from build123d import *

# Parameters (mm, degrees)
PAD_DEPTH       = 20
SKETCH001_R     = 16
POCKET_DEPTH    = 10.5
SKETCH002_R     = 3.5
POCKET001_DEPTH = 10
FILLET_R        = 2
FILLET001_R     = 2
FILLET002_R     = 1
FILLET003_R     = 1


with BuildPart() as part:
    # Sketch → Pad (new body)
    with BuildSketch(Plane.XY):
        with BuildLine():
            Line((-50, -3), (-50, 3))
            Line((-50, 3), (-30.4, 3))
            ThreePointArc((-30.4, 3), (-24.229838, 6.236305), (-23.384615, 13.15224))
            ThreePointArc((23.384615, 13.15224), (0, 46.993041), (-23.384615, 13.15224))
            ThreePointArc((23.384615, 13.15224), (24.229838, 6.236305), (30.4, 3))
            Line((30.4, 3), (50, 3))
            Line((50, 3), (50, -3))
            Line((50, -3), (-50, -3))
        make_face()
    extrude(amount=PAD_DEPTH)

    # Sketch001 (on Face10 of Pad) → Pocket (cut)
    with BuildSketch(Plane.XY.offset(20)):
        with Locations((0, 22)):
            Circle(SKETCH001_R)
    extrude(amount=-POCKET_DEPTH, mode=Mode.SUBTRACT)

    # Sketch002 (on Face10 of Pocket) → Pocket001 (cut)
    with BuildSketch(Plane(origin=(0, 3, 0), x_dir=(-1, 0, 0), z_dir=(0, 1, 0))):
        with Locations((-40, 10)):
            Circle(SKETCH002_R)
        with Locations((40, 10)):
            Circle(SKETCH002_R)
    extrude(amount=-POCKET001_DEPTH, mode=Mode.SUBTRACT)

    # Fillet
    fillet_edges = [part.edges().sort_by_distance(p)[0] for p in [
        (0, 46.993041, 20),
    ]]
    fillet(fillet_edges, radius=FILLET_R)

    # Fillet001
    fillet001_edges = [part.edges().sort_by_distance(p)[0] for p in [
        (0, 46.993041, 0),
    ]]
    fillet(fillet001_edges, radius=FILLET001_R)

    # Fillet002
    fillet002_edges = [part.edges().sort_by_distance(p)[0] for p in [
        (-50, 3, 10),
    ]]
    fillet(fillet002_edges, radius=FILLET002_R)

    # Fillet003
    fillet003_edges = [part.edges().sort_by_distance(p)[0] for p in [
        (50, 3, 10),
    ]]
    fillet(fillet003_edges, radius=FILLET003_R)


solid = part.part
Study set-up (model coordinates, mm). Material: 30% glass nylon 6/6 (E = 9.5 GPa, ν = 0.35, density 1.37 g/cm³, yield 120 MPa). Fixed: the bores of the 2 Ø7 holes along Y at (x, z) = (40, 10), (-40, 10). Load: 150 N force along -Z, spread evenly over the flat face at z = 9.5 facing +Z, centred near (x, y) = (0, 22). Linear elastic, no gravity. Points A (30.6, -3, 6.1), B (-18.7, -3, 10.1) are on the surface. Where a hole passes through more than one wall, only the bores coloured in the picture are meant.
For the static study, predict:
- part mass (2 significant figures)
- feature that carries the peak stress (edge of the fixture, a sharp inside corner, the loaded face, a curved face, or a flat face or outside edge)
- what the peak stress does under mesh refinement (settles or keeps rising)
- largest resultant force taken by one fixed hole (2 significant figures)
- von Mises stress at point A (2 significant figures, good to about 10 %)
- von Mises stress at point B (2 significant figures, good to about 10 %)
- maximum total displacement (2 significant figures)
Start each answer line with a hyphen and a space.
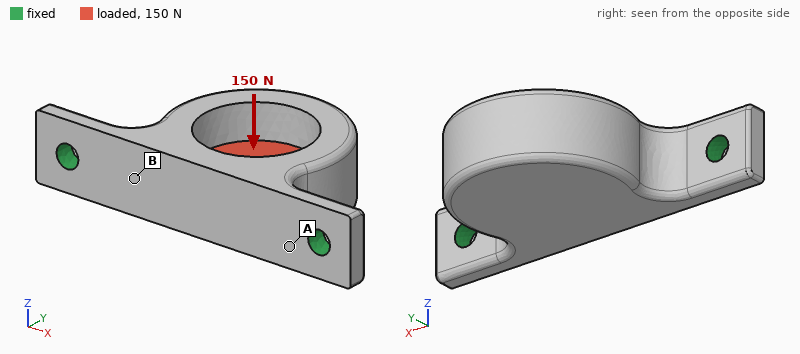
- 56 g
- edge of the fixture
- keeps rising
- 75 N
- 7.3 MPa
- 2.2 MPa
- 0.22 mm
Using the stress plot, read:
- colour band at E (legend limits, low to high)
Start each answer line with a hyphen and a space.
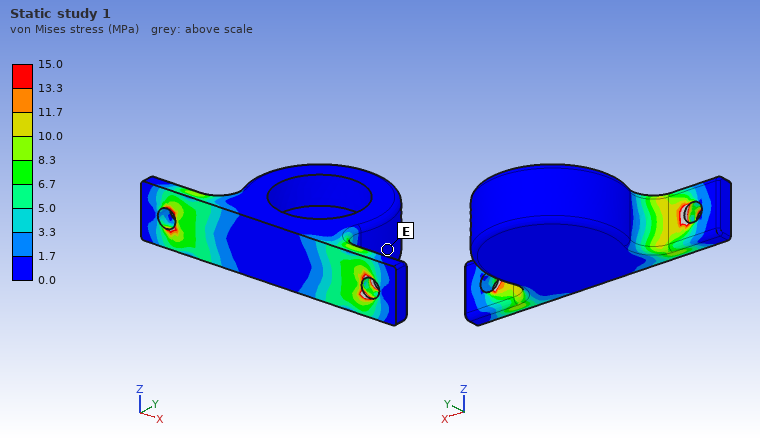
- 0.0 to 1.7 MPa
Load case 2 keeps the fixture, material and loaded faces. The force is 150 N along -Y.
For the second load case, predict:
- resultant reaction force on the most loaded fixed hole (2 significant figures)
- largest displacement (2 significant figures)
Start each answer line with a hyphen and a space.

- 93 N
- 13 µm
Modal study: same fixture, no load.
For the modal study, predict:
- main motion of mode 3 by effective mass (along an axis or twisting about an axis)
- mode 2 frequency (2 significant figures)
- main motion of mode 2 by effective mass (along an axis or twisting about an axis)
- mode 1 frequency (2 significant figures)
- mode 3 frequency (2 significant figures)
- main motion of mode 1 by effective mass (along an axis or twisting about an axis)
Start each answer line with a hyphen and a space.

- along X
- 2600 Hz
- along Y
- 780 Hz
- 2900 Hz
- along Z
